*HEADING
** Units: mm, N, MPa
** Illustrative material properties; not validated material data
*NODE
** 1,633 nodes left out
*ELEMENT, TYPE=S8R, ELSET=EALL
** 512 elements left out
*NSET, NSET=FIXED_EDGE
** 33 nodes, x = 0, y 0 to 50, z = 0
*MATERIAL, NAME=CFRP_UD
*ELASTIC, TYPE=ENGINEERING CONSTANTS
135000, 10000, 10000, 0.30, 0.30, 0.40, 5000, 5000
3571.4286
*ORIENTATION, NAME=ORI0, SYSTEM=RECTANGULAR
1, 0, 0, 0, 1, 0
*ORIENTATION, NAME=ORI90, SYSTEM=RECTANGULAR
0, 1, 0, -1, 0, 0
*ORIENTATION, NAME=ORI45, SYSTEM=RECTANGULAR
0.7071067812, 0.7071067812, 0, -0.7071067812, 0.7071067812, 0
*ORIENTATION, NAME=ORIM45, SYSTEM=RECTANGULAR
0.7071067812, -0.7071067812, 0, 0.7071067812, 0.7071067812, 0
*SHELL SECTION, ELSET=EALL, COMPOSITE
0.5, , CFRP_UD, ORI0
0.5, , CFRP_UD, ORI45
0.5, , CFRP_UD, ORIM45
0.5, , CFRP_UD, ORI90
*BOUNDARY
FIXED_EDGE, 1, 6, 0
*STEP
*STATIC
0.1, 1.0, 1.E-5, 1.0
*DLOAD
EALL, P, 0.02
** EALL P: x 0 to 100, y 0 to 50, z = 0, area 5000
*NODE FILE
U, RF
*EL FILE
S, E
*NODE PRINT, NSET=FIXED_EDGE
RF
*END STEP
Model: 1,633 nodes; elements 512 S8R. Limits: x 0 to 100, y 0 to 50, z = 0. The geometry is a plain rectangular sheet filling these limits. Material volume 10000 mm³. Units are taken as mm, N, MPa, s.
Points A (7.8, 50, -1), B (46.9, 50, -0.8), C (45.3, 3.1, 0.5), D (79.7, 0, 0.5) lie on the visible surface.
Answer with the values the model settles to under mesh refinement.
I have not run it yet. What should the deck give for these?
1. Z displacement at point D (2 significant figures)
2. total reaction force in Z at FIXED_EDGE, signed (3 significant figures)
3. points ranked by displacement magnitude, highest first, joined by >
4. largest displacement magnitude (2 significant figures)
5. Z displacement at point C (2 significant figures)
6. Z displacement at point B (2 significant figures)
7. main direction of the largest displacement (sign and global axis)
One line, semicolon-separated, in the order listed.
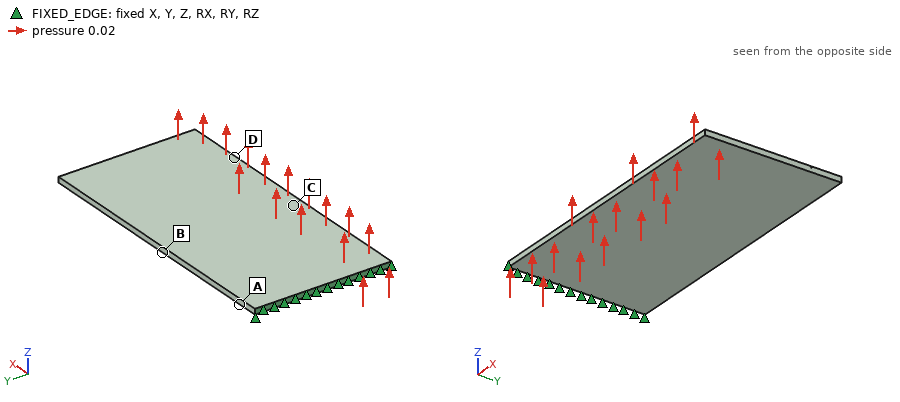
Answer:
7.4 mm; -100 N; D > B > C > A; 11 mm; 2.9 mm; 3.8 mm; +Z
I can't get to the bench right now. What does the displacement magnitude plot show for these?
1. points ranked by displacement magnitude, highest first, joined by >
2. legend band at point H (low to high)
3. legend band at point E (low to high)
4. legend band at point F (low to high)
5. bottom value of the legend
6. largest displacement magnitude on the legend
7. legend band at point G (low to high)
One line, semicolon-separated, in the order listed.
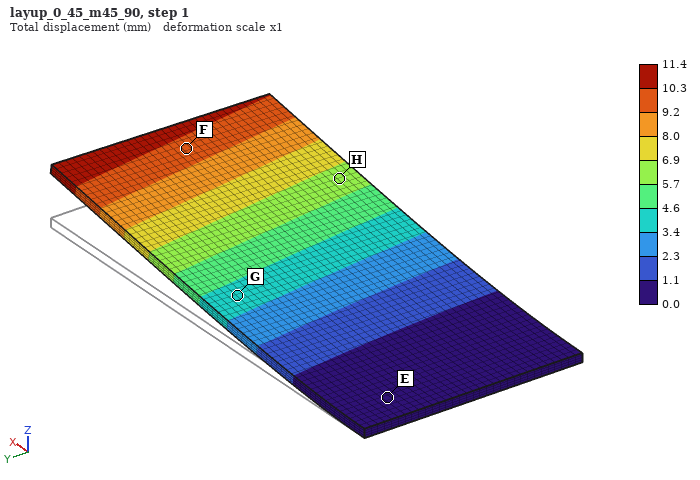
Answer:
F > H > G > E; 5.7 to 6.9 mm; 0.0 to 1.1 mm; 9.2 to 10.3 mm; 0.0 mm; 11.4 mm; 3.4 to 4.6 mm
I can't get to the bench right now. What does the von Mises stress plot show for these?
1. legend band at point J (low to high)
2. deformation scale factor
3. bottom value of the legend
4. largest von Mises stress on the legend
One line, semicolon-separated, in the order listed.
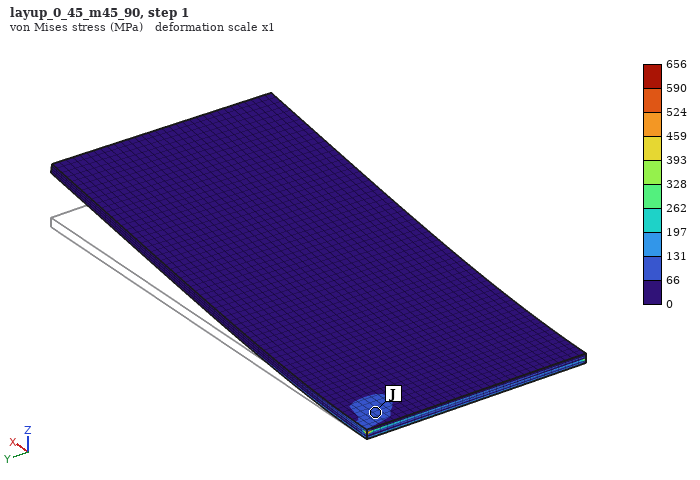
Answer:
66 to 131 MPa; 1; 0 MPa; 656 MPa
